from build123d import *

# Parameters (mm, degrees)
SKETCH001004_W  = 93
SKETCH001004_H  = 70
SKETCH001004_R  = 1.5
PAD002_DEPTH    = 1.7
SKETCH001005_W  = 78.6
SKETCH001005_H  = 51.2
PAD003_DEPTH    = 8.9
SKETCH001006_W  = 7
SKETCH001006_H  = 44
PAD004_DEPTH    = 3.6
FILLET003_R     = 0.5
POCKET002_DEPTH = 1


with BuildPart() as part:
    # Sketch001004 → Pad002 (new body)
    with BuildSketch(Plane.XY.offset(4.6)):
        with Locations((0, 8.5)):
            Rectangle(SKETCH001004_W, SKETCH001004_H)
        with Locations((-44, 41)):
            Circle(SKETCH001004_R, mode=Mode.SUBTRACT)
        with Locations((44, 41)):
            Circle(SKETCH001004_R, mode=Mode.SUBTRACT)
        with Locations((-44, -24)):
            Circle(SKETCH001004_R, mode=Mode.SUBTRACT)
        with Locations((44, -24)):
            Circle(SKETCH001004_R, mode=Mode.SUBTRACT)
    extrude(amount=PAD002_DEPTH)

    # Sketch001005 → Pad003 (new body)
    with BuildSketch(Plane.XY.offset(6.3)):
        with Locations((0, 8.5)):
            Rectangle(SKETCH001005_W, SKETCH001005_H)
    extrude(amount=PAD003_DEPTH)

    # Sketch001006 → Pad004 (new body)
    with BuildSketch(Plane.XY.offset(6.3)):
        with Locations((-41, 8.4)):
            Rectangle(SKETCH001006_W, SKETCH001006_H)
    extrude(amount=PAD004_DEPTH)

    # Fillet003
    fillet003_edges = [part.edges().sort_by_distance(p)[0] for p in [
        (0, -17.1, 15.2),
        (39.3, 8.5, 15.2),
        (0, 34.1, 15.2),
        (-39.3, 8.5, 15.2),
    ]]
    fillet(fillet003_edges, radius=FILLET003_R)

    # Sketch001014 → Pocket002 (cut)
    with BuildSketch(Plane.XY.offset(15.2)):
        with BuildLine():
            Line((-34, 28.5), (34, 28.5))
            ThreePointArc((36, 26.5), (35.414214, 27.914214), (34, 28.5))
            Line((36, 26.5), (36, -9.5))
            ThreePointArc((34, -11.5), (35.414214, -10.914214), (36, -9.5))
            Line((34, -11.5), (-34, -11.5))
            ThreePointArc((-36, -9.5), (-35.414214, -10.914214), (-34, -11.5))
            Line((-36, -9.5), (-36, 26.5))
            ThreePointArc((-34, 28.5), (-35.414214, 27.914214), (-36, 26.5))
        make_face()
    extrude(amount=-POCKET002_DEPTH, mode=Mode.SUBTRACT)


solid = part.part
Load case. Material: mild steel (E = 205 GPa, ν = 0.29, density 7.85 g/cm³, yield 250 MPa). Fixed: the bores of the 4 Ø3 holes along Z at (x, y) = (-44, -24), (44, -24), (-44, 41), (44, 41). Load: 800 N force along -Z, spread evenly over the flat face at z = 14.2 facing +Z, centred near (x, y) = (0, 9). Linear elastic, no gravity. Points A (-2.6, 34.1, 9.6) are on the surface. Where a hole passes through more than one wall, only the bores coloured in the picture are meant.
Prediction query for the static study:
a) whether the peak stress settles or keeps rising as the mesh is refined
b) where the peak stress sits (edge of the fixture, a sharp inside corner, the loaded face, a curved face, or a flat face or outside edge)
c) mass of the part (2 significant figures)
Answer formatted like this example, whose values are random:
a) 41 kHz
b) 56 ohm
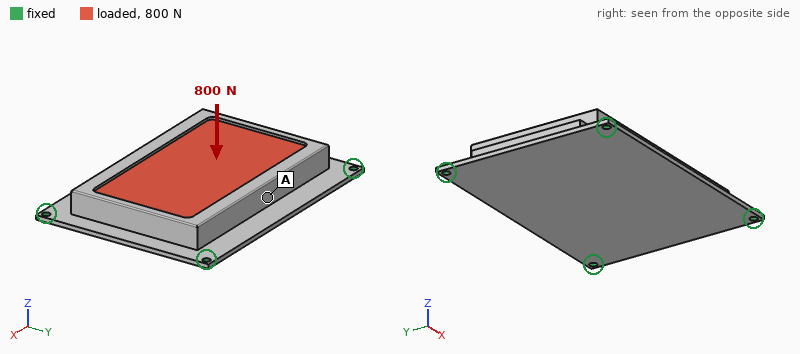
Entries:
a) keeps rising
b) edge of the fixture
c) 350 g
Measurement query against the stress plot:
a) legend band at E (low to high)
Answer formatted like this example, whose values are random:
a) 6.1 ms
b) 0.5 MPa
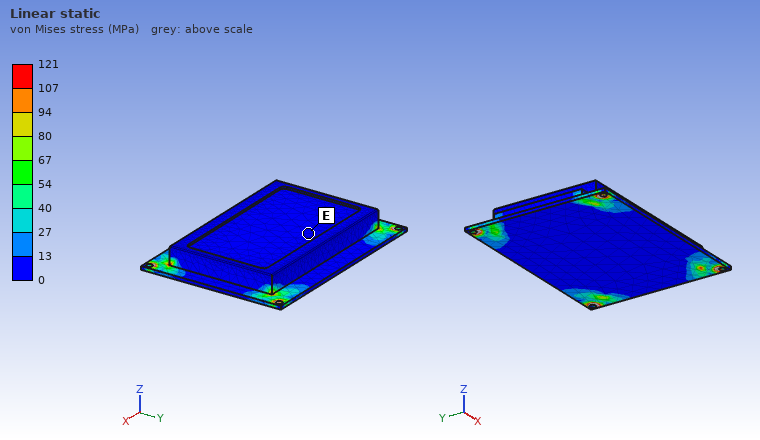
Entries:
a) 0 to 13 MPa
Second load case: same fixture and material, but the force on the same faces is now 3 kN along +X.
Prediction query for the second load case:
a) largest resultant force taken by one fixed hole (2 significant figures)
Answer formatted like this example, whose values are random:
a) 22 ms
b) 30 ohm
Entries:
a) 860 N
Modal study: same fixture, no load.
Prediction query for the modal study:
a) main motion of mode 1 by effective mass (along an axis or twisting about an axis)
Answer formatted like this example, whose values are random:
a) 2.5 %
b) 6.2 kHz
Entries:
a) along Z
